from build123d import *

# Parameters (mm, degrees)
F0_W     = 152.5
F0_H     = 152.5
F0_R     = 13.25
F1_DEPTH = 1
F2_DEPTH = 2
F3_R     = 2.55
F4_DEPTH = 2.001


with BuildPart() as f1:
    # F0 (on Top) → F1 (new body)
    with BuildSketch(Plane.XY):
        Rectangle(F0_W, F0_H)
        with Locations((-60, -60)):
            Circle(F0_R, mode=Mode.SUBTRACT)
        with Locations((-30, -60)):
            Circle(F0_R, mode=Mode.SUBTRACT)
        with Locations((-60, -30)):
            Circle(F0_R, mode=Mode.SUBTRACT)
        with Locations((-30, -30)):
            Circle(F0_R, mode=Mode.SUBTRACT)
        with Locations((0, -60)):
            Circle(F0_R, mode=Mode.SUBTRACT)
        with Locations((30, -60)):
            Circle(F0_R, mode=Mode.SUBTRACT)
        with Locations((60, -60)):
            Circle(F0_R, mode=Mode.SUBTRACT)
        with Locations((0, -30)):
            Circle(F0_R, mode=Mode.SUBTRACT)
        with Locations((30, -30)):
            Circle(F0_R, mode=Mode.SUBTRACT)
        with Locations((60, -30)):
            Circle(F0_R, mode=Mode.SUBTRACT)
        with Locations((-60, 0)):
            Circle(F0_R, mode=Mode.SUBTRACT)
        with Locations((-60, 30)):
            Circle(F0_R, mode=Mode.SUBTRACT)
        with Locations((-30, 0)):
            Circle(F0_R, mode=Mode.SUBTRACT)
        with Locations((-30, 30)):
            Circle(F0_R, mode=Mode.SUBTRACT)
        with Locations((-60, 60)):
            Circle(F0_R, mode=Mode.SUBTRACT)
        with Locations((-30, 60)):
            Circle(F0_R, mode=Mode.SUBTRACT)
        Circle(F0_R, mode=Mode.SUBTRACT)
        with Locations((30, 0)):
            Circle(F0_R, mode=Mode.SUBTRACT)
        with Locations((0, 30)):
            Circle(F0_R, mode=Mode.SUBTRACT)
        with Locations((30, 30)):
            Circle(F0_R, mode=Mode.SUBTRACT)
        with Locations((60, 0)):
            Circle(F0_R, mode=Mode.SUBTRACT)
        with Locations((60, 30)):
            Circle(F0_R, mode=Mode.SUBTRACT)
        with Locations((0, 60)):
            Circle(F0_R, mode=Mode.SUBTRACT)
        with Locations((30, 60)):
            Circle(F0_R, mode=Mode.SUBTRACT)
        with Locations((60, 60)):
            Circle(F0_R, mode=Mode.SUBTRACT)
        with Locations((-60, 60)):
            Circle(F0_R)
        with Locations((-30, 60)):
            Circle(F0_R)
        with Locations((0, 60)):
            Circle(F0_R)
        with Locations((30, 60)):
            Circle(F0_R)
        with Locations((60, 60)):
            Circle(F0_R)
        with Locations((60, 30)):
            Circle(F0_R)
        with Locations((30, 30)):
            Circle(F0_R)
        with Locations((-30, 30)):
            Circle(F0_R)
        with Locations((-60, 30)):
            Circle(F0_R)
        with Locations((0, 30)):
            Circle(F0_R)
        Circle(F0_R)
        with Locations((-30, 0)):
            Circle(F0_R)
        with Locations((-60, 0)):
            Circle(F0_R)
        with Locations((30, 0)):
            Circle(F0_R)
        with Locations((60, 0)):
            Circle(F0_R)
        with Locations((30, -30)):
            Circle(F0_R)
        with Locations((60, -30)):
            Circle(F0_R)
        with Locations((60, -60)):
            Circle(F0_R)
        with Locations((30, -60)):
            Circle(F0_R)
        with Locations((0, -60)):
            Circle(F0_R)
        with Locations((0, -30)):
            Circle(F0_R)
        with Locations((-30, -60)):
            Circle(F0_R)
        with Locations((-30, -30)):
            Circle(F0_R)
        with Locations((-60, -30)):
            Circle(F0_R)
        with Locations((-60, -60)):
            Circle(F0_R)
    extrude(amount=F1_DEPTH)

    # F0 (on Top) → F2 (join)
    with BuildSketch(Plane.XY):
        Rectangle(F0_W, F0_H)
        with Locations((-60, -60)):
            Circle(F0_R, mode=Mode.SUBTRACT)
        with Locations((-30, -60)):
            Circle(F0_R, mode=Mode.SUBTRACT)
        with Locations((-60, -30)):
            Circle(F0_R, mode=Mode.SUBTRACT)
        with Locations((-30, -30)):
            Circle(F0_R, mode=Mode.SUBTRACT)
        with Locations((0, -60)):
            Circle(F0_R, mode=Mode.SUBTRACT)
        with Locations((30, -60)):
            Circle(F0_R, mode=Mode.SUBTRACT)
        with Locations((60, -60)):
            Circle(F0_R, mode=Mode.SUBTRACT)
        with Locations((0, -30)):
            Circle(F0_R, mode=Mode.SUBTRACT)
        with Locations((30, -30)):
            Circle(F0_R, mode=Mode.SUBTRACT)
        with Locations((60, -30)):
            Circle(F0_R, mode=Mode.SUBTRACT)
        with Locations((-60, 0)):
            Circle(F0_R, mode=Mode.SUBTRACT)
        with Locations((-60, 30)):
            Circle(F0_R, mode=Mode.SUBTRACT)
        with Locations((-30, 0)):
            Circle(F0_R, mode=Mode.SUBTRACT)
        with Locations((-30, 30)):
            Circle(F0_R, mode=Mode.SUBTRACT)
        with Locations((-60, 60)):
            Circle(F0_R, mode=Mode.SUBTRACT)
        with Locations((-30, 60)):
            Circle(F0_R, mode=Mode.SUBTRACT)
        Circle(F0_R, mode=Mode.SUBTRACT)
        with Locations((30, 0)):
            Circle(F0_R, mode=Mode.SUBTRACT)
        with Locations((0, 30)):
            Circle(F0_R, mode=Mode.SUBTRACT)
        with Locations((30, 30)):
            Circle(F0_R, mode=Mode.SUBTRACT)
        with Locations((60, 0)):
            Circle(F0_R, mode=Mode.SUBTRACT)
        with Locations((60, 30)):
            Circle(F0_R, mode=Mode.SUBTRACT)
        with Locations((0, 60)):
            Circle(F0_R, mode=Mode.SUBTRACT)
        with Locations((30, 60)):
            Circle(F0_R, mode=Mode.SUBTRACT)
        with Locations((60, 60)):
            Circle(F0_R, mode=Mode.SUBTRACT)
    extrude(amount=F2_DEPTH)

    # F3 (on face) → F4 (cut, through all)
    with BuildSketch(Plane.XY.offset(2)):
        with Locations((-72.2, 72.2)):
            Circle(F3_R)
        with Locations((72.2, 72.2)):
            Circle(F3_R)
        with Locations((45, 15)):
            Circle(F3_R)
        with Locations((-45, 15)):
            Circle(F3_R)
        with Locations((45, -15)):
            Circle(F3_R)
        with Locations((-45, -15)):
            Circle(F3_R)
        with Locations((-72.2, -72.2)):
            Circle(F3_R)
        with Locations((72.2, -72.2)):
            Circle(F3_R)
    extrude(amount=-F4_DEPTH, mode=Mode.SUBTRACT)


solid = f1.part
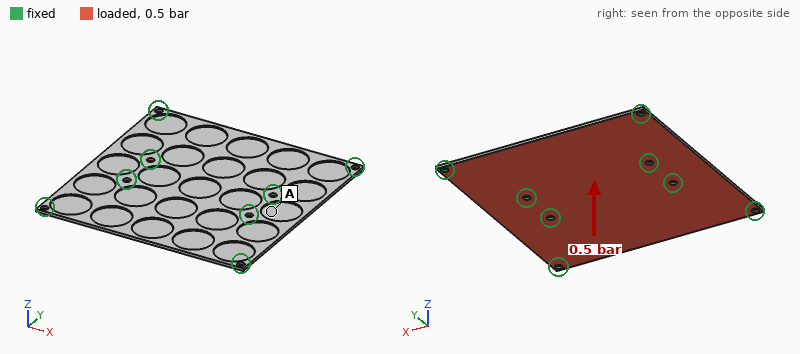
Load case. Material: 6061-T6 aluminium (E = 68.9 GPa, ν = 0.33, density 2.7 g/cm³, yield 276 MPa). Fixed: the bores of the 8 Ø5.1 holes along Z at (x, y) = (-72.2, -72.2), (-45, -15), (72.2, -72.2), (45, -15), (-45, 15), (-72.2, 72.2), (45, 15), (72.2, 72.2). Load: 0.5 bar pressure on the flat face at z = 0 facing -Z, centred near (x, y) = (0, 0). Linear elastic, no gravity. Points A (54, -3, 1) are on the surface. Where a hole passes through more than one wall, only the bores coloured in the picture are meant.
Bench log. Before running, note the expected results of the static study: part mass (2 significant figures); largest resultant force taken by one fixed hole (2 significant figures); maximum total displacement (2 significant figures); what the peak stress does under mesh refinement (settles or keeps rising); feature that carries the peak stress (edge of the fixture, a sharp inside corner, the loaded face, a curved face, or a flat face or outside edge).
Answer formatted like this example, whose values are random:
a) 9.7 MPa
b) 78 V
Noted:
a) 87 g
b) 260 N
c) 1.8 mm
d) keeps rising
e) edge of the fixture
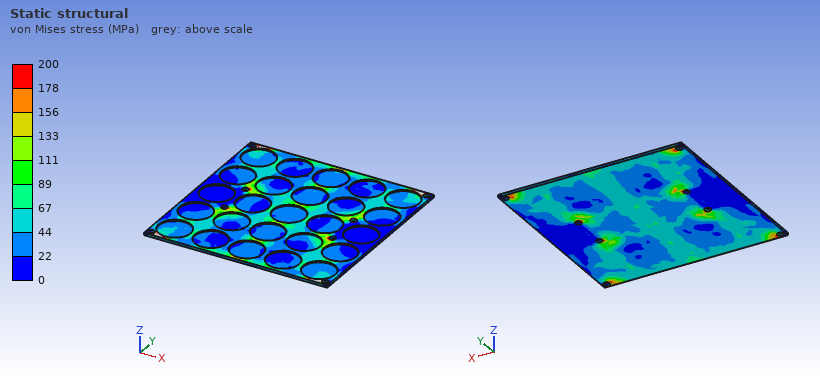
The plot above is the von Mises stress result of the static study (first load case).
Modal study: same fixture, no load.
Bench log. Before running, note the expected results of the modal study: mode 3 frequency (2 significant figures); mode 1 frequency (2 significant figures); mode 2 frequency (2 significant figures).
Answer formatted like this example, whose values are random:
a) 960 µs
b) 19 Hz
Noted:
a) 1200 Hz
b) 560 Hz
c) 570 Hz
